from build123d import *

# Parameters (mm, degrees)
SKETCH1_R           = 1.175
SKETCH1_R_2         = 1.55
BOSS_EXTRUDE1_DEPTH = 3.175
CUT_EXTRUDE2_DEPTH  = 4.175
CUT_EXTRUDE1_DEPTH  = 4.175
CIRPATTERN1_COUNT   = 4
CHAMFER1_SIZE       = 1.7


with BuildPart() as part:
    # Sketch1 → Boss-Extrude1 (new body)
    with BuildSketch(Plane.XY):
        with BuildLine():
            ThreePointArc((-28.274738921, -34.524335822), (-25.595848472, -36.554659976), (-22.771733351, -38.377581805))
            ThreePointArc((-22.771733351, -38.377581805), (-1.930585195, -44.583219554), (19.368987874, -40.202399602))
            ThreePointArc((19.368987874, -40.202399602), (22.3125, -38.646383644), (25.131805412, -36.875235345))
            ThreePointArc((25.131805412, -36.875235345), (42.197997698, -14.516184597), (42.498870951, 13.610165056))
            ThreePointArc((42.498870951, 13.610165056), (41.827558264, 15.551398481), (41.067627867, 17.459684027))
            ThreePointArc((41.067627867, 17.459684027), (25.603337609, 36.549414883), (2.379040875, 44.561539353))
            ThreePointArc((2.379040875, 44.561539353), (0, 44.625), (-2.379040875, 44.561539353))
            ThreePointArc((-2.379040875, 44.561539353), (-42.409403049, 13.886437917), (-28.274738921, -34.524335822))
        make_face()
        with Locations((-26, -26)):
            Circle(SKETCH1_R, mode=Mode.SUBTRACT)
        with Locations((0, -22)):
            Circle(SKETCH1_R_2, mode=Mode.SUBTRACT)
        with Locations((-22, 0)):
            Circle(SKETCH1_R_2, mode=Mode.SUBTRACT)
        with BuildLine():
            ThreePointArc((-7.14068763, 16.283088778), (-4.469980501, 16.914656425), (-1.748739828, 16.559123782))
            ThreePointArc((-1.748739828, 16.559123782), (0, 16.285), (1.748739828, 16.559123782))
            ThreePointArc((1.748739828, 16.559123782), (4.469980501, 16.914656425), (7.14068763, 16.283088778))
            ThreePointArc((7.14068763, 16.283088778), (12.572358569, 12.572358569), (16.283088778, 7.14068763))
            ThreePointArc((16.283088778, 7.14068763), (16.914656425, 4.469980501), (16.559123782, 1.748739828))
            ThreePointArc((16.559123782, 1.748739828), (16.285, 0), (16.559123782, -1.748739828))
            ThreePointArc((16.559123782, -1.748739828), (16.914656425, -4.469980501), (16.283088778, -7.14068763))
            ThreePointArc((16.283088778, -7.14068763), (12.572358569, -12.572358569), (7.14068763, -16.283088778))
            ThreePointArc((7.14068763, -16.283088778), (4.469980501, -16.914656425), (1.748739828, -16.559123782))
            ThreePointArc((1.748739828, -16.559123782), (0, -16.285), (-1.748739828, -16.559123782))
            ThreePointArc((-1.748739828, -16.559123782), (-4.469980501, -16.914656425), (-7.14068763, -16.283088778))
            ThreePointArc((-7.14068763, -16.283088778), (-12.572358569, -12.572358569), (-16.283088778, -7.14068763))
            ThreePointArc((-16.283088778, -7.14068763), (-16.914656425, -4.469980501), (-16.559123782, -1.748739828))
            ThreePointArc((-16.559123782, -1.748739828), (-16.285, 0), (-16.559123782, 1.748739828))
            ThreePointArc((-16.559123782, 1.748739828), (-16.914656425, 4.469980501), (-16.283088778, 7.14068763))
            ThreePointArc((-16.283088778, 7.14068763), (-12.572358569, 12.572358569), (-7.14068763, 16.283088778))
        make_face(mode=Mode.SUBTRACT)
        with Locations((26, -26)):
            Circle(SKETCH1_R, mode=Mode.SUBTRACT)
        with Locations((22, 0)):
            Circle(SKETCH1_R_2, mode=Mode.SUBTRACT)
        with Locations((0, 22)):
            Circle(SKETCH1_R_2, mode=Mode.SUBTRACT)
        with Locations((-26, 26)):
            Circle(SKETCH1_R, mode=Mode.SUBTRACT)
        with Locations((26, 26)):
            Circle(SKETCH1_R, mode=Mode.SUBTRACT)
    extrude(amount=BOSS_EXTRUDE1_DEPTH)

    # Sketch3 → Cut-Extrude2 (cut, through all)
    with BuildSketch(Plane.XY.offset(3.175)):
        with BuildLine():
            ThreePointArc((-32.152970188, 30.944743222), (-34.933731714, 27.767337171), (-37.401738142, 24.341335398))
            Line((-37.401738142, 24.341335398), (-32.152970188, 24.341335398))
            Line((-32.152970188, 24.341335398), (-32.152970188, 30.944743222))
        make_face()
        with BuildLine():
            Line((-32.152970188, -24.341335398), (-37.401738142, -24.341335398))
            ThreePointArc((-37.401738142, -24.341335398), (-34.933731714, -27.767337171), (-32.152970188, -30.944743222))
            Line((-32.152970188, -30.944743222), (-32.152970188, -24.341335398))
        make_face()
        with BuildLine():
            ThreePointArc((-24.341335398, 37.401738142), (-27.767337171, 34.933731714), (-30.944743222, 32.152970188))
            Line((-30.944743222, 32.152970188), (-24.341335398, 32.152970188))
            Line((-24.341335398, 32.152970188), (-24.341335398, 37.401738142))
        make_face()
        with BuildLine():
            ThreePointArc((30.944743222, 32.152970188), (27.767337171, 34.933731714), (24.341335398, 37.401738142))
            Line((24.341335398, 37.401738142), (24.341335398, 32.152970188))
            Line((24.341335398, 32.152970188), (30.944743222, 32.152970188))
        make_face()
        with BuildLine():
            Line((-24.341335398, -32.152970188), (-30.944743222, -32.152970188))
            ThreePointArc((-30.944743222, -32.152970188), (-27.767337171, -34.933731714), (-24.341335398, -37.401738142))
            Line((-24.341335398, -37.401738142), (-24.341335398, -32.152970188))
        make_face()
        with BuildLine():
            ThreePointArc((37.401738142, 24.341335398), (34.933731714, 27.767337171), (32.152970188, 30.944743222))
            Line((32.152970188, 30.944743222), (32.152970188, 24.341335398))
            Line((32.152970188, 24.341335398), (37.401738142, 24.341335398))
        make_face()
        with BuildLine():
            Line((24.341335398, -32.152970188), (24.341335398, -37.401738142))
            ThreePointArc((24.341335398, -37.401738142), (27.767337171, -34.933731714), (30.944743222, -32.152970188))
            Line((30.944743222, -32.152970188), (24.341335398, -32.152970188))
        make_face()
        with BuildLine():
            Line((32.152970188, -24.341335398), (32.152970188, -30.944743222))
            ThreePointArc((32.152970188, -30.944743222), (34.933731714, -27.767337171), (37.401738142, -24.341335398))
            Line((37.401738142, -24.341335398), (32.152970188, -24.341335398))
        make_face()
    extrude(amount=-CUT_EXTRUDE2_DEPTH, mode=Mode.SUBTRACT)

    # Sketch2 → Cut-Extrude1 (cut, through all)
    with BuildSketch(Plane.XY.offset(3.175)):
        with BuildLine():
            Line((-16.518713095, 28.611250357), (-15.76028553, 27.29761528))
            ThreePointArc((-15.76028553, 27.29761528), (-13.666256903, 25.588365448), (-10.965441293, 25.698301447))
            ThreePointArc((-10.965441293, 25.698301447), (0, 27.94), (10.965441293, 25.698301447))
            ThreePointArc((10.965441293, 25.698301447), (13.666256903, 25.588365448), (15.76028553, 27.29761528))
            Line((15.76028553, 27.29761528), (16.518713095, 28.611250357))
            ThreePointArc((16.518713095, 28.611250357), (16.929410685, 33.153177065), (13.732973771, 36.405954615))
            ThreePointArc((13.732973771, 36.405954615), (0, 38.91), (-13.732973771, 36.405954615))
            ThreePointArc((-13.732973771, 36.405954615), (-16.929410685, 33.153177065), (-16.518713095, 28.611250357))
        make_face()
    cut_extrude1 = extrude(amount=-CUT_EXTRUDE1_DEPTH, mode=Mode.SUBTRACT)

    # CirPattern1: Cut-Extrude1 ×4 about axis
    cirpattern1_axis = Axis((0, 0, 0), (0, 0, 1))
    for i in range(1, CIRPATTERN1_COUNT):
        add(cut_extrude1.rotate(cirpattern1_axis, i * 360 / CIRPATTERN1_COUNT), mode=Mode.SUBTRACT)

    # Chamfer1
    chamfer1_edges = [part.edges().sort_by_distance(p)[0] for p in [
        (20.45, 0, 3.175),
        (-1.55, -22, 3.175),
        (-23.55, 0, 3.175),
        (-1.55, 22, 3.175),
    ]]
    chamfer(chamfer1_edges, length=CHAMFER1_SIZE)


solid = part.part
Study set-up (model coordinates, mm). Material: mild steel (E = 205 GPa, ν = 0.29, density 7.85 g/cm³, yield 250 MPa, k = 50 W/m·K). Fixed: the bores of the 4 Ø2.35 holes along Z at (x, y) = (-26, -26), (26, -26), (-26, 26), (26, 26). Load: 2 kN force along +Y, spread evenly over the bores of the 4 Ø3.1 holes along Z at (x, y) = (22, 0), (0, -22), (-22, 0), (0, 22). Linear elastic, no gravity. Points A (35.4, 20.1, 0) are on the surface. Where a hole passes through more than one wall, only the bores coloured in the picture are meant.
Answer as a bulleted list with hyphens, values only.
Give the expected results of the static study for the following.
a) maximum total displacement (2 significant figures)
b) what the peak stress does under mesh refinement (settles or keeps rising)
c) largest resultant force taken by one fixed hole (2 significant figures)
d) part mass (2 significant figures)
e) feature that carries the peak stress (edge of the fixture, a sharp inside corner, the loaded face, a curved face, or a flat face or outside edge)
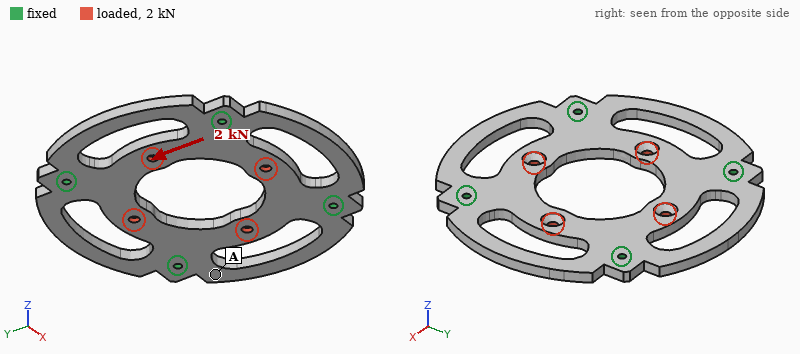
- 6.7 µm
- keeps rising
- 520 N
- 90 g
- edge of the fixture
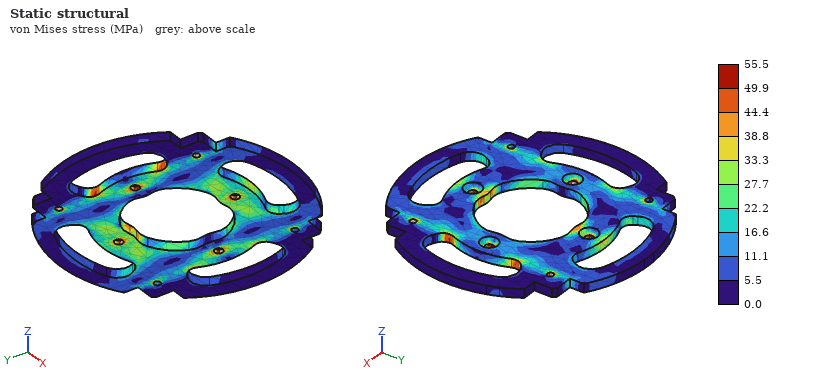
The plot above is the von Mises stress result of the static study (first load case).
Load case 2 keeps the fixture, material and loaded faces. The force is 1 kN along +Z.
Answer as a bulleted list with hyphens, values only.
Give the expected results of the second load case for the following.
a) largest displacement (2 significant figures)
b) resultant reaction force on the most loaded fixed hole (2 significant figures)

- 50 µm
- 260 N
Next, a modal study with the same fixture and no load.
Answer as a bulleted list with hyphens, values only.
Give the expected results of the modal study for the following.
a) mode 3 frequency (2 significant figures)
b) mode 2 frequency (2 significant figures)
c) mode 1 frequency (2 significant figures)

- 4300 Hz
- 4300 Hz
- 4000 Hz
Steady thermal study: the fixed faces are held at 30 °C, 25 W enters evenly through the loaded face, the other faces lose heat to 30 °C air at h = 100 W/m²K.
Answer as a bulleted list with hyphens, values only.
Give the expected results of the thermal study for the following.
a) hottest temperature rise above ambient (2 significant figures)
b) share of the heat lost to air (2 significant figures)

- 45 K
- 50 %
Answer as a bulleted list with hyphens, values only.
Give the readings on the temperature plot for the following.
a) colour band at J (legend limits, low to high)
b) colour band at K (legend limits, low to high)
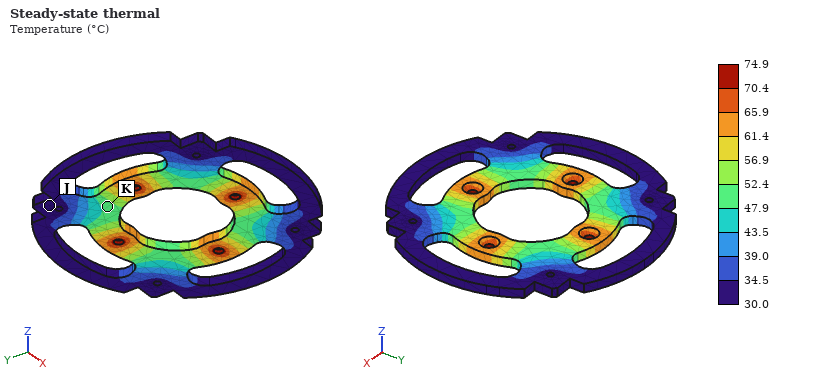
- 30.0 to 34.5 °C
- 47.9 to 52.4 °C
